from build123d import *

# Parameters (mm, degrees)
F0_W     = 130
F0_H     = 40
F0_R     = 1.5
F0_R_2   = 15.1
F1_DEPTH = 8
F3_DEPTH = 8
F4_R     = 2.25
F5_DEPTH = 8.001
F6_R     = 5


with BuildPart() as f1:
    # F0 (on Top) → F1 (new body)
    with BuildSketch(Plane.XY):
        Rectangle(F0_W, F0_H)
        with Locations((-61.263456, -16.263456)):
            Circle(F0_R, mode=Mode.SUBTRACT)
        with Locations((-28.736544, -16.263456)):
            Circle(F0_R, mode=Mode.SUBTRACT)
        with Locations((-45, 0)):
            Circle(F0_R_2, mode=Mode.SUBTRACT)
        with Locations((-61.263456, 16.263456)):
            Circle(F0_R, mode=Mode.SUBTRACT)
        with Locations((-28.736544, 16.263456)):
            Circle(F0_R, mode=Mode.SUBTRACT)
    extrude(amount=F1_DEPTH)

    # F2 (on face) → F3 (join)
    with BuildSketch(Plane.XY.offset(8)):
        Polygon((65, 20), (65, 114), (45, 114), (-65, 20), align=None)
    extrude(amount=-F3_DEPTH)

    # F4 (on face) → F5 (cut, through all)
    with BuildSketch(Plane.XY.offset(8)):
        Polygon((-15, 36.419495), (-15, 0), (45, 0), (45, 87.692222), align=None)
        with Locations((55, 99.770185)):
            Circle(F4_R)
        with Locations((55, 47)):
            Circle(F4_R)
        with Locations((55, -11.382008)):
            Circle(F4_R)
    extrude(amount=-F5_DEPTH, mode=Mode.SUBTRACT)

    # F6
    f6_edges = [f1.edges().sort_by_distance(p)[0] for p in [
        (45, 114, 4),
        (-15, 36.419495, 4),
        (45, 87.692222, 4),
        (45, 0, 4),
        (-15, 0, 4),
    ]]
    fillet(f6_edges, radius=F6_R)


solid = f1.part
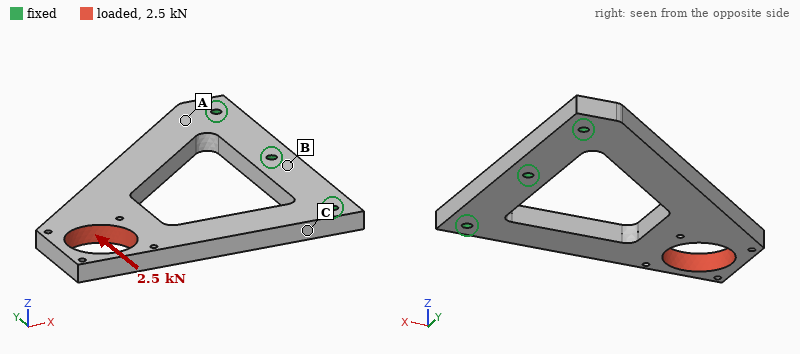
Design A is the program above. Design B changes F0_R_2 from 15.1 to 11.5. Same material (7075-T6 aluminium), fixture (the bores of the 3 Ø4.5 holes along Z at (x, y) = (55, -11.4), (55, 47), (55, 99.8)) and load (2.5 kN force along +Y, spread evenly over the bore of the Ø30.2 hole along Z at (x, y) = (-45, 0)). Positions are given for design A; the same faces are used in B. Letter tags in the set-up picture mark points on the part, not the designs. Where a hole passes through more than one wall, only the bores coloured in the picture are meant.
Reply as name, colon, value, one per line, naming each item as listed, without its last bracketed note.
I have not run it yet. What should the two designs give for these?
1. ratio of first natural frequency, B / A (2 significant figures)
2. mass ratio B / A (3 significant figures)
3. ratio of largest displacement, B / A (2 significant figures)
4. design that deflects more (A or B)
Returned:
ratio of first natural frequency, B / A: 0.93
mass ratio B / A: 1.04
ratio of largest displacement, B / A: 0.81
design that deflects more: A
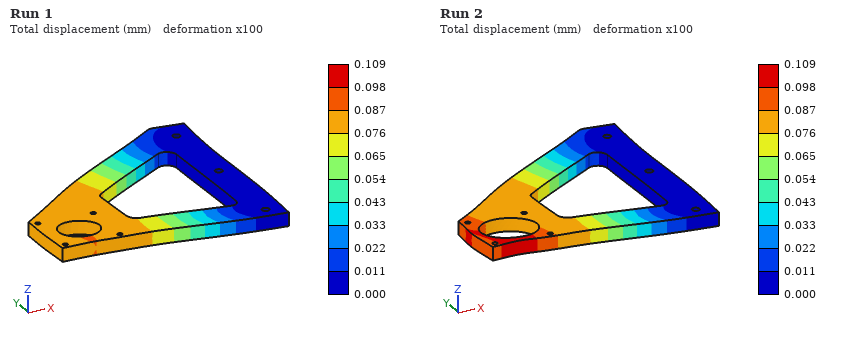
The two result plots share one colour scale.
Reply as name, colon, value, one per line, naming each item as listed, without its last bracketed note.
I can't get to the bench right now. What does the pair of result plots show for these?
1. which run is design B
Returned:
which run is design B: Run 1
